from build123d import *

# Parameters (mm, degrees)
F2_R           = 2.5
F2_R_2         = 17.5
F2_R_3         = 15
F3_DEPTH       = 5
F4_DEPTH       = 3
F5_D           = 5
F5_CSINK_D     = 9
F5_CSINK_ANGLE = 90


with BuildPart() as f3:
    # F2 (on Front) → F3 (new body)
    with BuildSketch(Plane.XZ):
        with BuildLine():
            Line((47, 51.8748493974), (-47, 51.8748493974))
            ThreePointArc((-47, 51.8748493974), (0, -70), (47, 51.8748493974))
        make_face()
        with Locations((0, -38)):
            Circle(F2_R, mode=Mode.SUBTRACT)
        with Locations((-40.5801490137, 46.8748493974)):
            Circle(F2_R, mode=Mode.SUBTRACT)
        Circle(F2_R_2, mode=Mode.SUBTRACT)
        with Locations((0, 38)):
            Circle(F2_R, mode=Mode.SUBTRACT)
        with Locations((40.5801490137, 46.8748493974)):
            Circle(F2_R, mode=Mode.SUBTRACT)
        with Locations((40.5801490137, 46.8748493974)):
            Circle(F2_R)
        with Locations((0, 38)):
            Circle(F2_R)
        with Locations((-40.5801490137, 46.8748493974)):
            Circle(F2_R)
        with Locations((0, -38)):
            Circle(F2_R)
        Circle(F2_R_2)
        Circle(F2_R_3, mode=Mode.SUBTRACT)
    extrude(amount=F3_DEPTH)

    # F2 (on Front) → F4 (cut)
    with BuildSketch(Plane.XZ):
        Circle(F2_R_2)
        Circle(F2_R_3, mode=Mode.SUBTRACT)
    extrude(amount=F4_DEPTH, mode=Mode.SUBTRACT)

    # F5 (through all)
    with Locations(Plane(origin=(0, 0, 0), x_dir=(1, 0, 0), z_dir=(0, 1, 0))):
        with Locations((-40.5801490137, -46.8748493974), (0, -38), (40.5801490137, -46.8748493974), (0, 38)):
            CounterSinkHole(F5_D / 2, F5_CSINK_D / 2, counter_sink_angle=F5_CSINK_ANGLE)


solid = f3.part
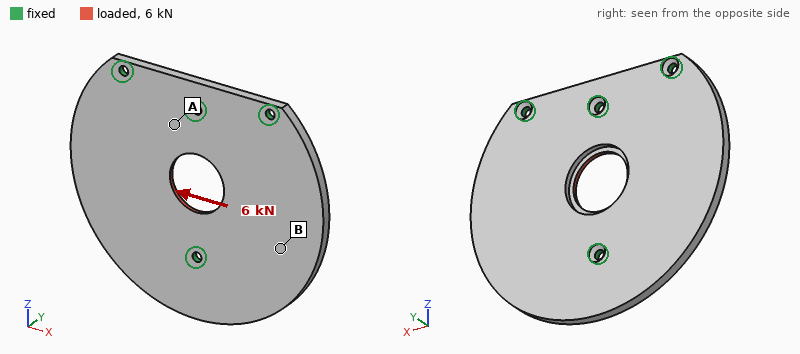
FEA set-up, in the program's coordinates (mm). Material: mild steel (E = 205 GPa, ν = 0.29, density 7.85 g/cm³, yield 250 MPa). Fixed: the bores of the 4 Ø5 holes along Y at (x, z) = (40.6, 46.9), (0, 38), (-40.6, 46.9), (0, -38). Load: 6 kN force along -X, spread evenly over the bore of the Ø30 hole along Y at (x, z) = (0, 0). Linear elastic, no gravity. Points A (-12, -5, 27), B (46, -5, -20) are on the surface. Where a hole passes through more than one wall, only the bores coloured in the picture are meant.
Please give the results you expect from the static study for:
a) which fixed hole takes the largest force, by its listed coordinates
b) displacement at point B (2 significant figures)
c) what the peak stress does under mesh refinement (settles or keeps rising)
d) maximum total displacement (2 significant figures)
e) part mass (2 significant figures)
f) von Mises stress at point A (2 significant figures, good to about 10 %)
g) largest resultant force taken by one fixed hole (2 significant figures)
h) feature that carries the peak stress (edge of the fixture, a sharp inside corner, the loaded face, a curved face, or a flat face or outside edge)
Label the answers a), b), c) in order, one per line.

a) (0, -38)
b) 10.0 µm
c) keeps rising
d) 14 µm
e) 520 g
f) 17 MPa
g) 2.9 kN
h) edge of the fixture
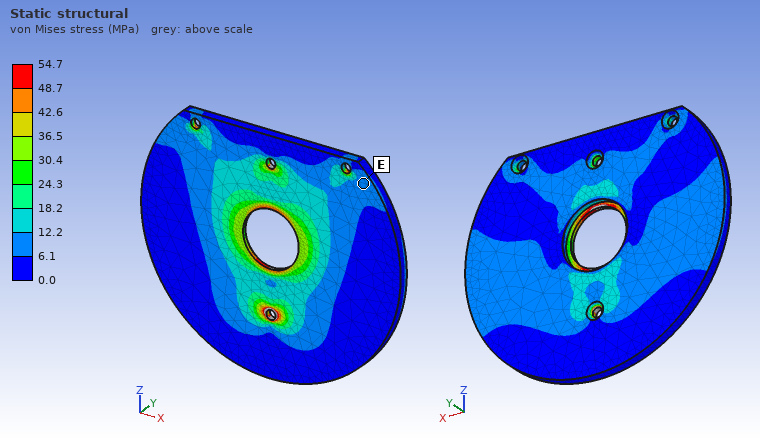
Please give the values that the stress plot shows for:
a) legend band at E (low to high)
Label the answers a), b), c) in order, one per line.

a) 6.1 to 12.2 MPa
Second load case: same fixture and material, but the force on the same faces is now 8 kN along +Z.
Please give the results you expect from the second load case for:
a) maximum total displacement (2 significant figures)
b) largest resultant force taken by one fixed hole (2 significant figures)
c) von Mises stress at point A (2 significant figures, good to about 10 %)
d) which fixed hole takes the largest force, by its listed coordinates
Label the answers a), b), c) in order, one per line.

a) 5.1 µm
b) 3.0 kN
c) 19 MPa
d) (0, -38)
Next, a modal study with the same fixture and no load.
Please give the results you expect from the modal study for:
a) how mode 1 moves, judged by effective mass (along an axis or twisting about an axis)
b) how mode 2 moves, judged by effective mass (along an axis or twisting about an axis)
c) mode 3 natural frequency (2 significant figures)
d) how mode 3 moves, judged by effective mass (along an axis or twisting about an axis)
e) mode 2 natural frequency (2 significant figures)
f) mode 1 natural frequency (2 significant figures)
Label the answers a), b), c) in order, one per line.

a) twisting about Z
b) along Y
c) 2600 Hz
d) twisting about X
e) 1300 Hz
f) 1100 Hz
